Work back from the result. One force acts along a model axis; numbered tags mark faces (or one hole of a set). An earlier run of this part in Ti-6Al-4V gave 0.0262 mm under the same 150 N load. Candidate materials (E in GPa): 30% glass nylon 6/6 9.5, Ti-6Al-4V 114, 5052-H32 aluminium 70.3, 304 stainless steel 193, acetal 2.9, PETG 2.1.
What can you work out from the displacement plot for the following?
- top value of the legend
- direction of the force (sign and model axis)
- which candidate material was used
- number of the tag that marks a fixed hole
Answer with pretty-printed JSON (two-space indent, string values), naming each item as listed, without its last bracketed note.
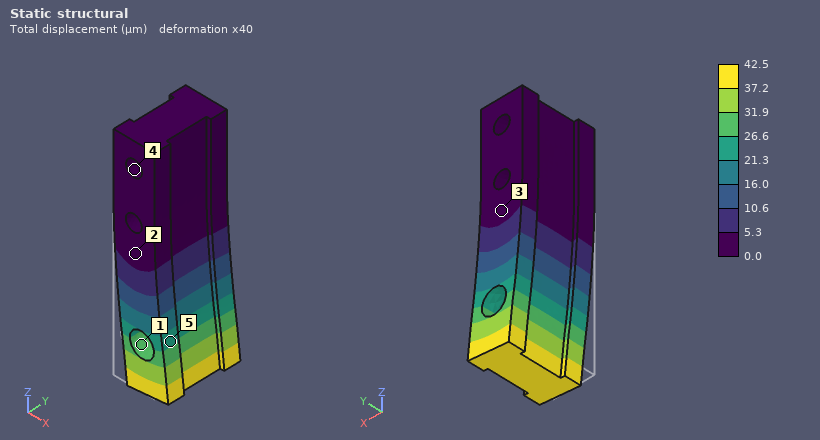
{
  "top value of the legend": "42.5 µm",
  "direction of the force": "+X",
  "which candidate material was used": "5052-H32 aluminium",
  "number of the tag that marks a fixed hole": "4"
}
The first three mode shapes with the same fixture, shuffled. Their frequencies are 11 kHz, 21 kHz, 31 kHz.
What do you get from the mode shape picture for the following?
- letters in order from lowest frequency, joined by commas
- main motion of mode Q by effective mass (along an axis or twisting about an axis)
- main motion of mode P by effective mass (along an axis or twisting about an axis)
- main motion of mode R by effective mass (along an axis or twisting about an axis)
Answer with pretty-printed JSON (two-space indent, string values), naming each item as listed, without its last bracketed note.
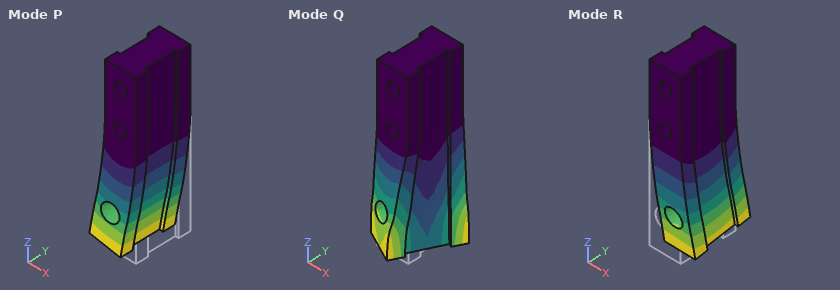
{
  "letters in order from lowest frequency, joined by commas": "P, R, Q",
  "main motion of mode Q by effective mass": "twisting about Z",
  "main motion of mode P by effective mass": "along X",
  "main motion of mode R by effective mass": "along Y"
}
